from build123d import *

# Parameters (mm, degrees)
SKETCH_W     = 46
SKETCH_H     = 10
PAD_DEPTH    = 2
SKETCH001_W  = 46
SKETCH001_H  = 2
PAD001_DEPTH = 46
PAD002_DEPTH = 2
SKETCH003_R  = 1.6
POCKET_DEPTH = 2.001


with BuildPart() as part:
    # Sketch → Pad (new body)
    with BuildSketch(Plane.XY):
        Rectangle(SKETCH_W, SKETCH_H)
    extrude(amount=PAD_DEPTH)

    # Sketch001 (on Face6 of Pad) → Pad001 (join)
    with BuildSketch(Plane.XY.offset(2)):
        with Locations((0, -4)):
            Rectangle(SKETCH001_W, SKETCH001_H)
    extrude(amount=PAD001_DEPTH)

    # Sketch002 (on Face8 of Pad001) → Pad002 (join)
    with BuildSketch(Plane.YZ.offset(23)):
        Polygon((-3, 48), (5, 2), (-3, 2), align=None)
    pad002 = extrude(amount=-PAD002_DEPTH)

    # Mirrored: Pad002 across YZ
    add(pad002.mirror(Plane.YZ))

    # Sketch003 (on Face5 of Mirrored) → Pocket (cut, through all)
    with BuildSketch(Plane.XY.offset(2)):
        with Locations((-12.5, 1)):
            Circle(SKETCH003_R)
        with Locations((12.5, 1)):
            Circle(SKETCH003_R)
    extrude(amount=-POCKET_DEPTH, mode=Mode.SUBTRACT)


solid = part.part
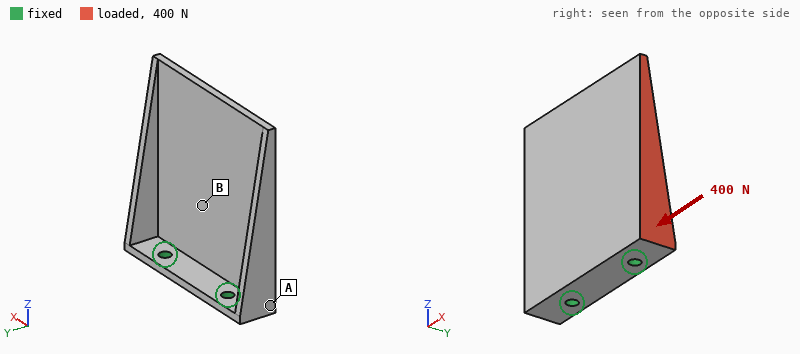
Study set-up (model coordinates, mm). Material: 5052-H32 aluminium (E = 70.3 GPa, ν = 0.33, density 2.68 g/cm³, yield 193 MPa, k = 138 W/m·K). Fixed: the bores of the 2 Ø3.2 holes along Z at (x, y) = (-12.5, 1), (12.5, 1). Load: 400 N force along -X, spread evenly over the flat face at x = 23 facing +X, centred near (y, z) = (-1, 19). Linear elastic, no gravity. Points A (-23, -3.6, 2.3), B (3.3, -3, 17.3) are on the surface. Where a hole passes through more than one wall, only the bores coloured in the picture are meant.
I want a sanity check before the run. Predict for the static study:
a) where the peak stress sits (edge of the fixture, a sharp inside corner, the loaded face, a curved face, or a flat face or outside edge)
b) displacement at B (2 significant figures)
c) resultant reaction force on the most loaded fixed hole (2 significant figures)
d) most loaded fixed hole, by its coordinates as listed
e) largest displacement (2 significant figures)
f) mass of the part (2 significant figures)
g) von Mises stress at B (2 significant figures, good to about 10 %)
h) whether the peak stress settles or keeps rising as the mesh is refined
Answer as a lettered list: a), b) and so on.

a) edge of the fixture
b) 0.021 mm
c) 370 N
d) (12.5, 1)
e) 0.11 mm
f) 16 g
g) 15 MPa
h) keeps rising
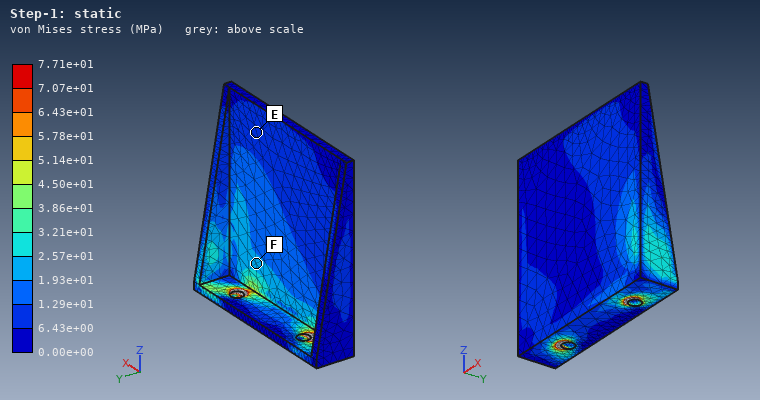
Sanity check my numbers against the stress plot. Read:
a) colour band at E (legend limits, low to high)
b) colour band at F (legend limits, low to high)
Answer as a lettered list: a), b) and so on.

a) 6.43e+00 to 1.29e+01 MPa
b) 1.93e+01 to 2.57e+01 MPa
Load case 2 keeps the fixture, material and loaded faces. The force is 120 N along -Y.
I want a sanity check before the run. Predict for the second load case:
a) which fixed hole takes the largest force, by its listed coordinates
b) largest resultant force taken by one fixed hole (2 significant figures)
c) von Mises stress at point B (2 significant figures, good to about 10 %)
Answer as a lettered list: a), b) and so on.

a) (12.5, 1)
b) 160 N
c) 17 MPa
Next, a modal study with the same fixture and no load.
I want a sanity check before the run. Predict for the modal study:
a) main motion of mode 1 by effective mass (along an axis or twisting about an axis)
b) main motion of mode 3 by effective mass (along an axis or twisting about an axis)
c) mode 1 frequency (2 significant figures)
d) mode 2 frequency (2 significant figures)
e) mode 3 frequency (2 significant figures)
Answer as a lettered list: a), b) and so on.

a) along Y
b) along X
c) 950 Hz
d) 1900 Hz
e) 4500 Hz
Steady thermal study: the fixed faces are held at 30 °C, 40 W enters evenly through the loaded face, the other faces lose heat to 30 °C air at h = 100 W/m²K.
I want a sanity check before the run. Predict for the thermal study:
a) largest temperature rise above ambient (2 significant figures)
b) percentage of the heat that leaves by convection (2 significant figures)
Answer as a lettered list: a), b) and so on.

a) 66 K
b) 38 %
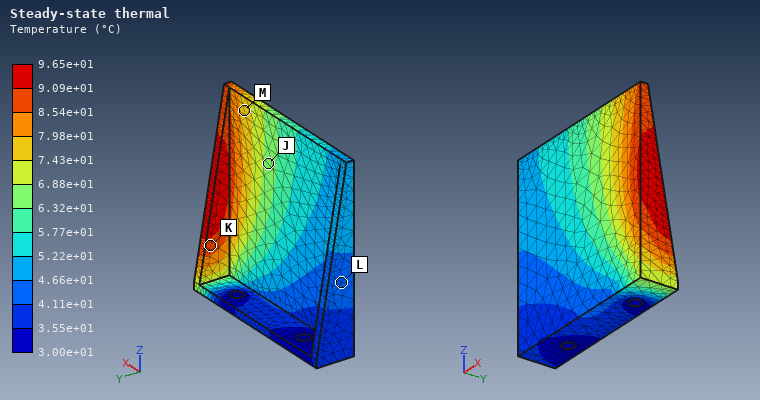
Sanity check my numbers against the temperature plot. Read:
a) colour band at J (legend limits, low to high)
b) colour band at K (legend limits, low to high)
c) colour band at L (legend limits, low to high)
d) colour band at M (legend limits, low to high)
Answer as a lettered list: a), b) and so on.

a) 6.32e+01 to 6.88e+01 °C
b) 8.54e+01 to 9.09e+01 °C
c) 4.11e+01 to 4.66e+01 °C
d) 7.43e+01 to 7.98e+01 °C
